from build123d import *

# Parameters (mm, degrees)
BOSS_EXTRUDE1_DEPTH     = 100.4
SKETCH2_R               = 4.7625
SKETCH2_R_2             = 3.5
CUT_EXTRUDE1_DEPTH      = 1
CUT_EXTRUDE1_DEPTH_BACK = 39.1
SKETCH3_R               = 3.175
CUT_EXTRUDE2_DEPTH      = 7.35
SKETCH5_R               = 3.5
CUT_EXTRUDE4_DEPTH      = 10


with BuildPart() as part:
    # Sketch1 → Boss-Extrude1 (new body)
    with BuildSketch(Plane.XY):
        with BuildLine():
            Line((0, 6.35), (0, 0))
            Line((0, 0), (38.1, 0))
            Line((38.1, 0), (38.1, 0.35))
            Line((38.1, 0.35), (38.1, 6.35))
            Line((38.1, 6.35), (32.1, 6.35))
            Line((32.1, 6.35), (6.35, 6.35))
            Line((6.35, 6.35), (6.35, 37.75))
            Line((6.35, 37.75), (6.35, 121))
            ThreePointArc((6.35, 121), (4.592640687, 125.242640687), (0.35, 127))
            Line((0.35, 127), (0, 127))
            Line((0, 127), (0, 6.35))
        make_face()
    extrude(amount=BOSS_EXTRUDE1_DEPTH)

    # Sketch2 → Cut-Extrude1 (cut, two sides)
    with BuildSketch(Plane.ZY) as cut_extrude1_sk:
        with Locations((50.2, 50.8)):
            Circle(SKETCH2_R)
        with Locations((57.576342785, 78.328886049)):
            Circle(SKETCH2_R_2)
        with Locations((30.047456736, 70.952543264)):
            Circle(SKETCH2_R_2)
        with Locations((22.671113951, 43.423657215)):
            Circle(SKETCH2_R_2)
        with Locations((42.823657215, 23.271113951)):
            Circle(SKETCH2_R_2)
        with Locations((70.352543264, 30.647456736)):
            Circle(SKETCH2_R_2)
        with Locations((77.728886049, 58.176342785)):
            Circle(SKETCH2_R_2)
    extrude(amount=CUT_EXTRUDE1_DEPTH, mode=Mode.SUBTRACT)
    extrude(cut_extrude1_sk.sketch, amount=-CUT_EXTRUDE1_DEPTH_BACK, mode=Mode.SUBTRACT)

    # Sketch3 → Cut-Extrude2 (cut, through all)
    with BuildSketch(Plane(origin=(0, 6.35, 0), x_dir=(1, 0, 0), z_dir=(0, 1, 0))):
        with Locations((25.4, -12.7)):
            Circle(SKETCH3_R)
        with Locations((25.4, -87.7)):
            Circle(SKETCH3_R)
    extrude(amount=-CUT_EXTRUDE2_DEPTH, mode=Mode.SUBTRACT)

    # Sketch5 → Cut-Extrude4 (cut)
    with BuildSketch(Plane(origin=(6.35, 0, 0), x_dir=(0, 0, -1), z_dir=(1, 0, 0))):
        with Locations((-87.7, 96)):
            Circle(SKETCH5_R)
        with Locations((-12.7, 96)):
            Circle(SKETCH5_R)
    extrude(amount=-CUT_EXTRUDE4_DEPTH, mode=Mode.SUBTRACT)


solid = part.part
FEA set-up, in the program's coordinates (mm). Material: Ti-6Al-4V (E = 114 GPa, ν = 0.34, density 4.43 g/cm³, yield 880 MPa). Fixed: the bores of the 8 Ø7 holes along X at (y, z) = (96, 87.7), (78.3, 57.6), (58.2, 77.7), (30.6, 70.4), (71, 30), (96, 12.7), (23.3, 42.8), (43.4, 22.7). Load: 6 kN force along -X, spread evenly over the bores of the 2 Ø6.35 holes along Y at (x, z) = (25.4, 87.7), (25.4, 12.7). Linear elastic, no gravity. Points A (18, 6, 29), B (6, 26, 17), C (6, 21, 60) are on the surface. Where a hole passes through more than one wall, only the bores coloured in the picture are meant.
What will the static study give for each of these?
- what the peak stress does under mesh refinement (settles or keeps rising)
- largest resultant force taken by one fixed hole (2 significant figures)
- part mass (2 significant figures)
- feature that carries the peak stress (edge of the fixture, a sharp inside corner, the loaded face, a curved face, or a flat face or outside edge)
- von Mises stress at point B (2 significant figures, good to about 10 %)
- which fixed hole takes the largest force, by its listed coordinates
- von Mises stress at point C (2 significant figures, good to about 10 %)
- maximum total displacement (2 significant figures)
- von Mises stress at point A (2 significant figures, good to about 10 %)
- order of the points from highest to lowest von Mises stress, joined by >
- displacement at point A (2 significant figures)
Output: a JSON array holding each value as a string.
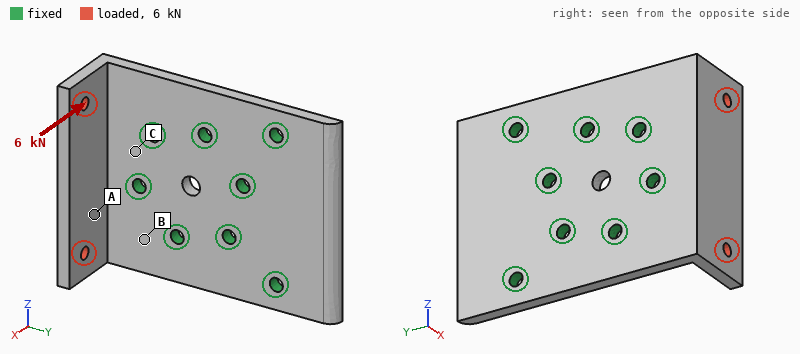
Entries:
["keeps rising", "5.4 kN", "430 g", "edge of the fixture", "69 MPa", "(23.3, 42.8)", "120 MPa", "0.28 mm", "33 MPa", "C > B > A", "0.13 mm"]
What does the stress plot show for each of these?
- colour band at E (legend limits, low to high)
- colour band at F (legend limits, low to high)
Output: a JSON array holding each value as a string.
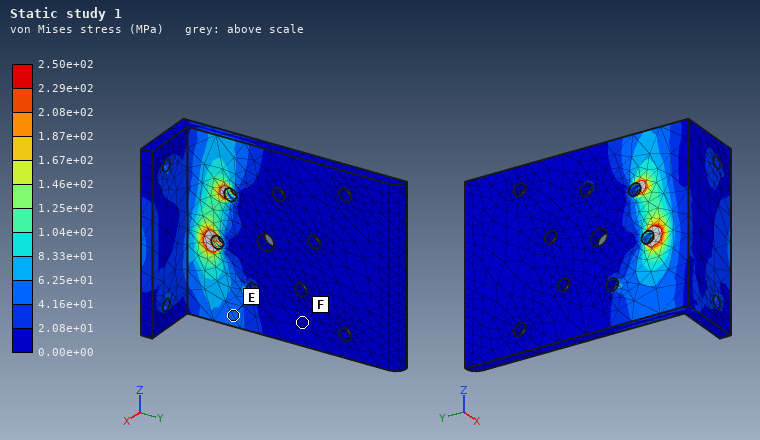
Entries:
["4.16e+01 to 6.25e+01 MPa", "0.00e+00 to 2.08e+01 MPa"]
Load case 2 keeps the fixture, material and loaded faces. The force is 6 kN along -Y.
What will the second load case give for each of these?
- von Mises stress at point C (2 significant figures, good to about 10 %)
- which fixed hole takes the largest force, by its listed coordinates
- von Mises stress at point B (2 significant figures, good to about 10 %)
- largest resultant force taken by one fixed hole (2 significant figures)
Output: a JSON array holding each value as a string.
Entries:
["150 MPa", "(23.3, 42.8)", "110 MPa", "3.3 kN"]
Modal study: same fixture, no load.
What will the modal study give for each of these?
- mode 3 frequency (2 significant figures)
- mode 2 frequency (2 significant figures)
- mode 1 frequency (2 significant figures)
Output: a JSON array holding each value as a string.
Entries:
["4300 Hz", "2400 Hz", "2100 Hz"]
